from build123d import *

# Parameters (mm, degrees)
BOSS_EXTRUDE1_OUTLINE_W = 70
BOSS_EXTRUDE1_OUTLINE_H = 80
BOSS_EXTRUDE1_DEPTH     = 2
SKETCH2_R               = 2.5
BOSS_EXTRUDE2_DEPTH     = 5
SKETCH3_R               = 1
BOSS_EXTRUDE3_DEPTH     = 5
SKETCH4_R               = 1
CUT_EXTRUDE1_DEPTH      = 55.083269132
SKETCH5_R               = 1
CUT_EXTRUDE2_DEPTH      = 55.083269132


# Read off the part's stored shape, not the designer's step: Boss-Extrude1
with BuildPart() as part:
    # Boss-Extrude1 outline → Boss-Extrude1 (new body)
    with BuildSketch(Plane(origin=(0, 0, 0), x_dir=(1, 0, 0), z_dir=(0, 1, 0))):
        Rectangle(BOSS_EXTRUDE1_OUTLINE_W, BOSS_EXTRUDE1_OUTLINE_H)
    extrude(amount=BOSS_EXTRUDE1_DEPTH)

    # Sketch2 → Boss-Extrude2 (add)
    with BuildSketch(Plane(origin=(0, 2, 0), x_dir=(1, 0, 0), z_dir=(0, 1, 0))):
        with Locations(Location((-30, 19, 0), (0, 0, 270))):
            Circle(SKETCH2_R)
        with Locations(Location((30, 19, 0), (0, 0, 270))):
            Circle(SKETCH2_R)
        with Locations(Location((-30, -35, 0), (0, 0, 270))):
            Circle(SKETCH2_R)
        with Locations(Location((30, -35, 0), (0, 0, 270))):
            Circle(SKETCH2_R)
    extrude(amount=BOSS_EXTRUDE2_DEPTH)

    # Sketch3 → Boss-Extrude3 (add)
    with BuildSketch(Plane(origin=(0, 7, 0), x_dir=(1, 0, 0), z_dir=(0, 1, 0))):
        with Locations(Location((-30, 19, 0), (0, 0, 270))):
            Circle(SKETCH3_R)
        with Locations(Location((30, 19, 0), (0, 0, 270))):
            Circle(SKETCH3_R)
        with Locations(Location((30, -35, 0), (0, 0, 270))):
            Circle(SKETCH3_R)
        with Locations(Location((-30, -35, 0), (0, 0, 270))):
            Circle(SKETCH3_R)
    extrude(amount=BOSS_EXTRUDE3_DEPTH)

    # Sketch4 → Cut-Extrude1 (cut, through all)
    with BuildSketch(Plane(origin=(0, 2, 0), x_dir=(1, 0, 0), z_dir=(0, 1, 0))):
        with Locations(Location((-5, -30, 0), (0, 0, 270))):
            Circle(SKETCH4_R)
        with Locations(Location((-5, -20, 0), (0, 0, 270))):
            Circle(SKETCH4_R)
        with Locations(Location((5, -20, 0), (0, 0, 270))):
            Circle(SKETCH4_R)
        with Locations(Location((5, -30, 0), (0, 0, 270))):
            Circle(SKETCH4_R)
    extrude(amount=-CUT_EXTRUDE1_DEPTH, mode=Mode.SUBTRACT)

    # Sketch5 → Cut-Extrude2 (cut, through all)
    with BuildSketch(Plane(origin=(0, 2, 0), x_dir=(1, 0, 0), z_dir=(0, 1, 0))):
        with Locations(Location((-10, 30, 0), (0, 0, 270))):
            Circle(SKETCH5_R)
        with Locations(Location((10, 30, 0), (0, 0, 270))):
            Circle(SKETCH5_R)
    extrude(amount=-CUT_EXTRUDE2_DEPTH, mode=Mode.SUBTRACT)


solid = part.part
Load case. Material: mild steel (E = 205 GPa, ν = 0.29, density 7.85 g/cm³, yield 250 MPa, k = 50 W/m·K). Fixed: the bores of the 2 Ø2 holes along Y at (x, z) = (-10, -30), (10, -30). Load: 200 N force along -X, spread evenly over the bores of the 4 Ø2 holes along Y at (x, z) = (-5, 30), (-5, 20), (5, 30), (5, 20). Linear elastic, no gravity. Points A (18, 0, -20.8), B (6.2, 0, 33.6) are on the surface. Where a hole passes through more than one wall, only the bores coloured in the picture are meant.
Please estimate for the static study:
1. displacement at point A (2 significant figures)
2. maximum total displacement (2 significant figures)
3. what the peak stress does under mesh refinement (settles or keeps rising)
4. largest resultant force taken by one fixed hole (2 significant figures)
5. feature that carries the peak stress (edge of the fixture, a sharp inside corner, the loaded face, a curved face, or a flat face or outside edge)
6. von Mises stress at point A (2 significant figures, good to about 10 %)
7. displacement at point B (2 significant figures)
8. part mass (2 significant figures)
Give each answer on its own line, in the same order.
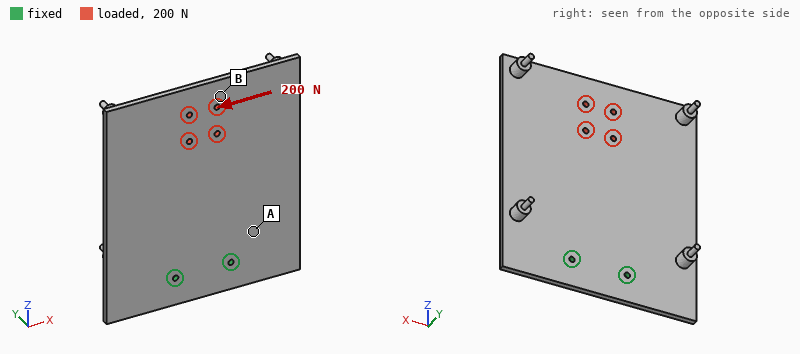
2.7 µm
13 µm
keeps rising
530 N
edge of the fixture
6.2 MPa
11 µm
91 g
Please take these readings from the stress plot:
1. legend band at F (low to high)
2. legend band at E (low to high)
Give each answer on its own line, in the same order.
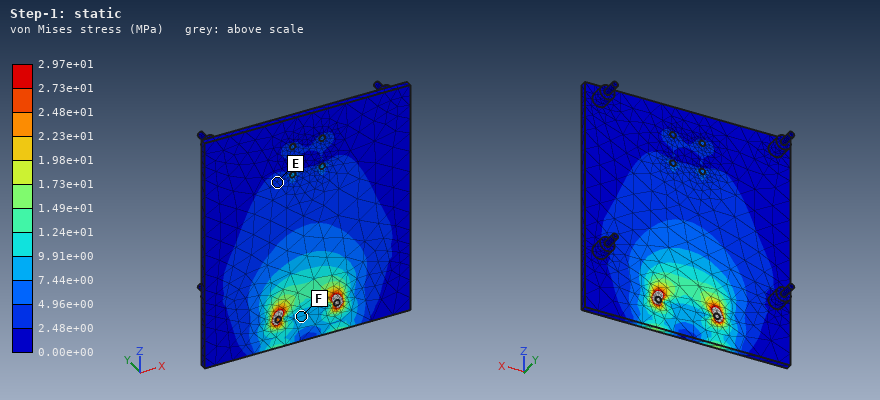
7.44e+00 to 9.91e+00 MPa
2.48e+00 to 4.96e+00 MPa
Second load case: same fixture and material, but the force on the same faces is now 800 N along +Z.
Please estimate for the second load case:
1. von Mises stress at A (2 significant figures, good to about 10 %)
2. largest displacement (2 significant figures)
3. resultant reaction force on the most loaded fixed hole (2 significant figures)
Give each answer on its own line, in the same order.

6.7 MPa
3.3 µm
400 N
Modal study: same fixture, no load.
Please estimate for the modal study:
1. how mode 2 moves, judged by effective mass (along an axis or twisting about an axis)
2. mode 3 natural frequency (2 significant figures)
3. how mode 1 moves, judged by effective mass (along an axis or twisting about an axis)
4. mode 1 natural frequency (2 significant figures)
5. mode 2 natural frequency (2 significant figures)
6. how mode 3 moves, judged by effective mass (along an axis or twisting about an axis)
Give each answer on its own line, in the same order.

twisting about Z
1600 Hz
along Y
290 Hz
650 Hz
along Y
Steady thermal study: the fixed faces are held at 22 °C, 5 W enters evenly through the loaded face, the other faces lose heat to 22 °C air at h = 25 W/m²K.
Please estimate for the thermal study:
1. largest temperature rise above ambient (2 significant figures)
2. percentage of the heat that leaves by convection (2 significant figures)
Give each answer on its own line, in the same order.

29 K
69 %
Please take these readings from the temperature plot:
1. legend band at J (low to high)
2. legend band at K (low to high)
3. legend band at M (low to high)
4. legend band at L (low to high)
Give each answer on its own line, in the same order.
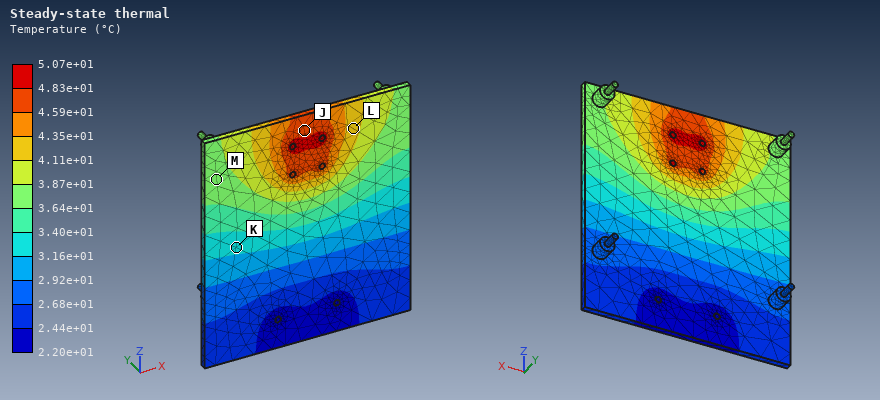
4.59e+01 to 4.83e+01 °C
3.16e+01 to 3.40e+01 °C
3.64e+01 to 3.87e+01 °C
4.11e+01 to 4.35e+01 °C
